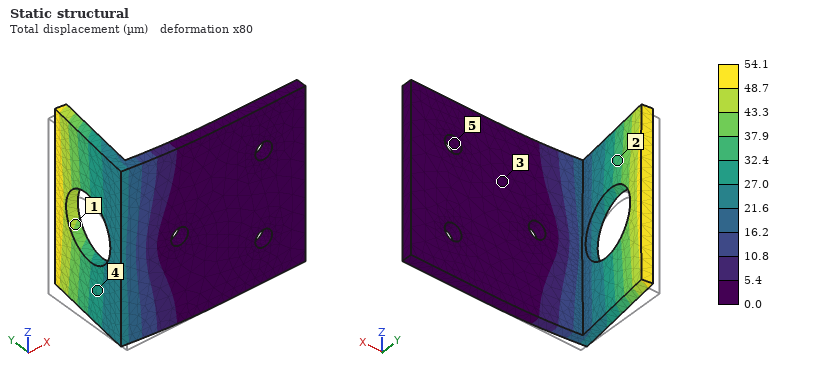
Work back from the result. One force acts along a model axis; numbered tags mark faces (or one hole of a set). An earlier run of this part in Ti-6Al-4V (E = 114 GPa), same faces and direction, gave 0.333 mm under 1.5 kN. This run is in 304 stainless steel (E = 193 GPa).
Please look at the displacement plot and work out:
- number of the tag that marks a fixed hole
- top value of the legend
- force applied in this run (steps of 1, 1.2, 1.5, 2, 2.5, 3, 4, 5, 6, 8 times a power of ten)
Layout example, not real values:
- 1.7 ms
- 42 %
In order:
- 5
- 54.1 µm
- 400 N
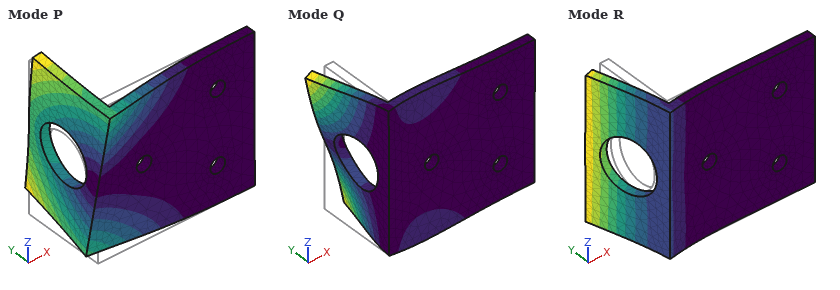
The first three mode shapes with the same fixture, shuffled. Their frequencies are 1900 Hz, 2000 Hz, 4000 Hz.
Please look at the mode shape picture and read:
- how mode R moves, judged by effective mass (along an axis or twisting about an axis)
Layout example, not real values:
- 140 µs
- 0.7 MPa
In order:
- along X
